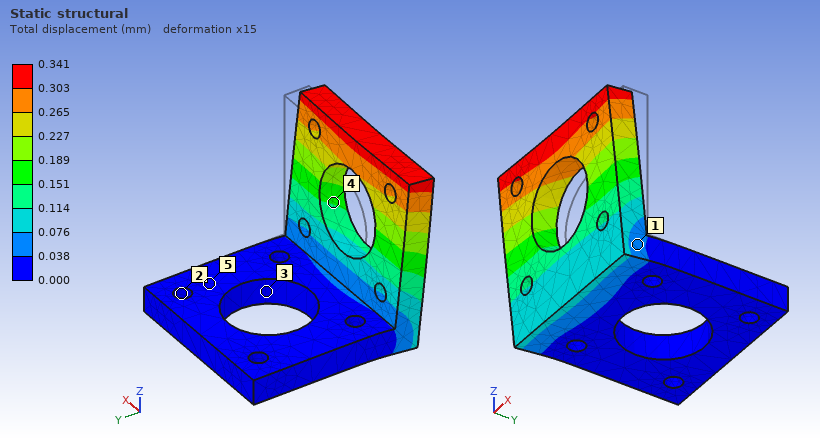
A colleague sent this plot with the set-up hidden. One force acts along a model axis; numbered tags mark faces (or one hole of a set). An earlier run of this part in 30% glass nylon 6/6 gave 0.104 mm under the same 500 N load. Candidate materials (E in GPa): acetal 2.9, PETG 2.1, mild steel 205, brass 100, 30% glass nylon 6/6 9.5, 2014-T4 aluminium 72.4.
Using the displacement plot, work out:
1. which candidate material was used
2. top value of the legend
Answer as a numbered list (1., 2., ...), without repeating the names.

1. acetal
2. 0.341 mm
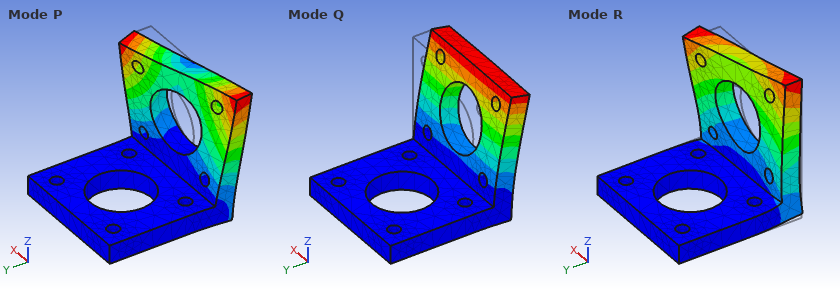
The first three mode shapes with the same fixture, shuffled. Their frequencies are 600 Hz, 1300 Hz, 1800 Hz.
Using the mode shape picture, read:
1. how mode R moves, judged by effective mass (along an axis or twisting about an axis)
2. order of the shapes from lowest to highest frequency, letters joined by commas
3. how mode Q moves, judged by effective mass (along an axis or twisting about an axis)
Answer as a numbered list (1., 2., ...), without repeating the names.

1. along X
2. Q, P, R
3. along Y
